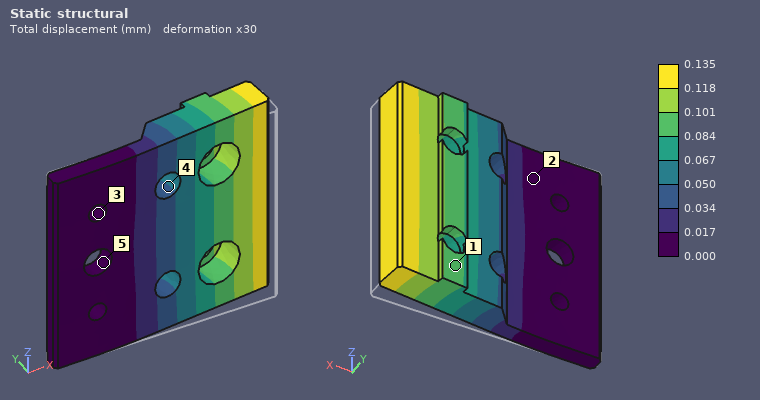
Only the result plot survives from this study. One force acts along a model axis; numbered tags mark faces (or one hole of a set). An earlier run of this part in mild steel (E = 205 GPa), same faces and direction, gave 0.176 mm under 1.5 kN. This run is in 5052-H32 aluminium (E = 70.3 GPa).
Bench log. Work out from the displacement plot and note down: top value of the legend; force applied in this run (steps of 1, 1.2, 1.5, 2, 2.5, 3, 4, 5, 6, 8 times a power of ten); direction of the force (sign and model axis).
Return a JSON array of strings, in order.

["0.135 mm", "400 N", "+Y"]
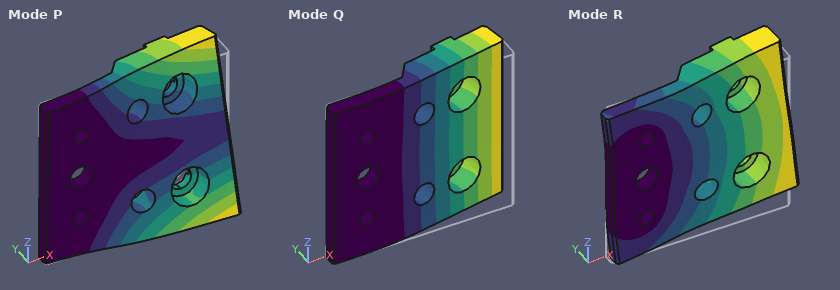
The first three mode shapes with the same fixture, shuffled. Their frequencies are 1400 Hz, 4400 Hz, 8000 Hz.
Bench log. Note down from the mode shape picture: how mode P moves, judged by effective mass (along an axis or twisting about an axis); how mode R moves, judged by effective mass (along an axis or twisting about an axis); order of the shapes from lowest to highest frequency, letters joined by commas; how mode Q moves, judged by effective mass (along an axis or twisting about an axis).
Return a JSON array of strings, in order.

["twisting about X", "along Z", "Q, P, R", "along Y"]
